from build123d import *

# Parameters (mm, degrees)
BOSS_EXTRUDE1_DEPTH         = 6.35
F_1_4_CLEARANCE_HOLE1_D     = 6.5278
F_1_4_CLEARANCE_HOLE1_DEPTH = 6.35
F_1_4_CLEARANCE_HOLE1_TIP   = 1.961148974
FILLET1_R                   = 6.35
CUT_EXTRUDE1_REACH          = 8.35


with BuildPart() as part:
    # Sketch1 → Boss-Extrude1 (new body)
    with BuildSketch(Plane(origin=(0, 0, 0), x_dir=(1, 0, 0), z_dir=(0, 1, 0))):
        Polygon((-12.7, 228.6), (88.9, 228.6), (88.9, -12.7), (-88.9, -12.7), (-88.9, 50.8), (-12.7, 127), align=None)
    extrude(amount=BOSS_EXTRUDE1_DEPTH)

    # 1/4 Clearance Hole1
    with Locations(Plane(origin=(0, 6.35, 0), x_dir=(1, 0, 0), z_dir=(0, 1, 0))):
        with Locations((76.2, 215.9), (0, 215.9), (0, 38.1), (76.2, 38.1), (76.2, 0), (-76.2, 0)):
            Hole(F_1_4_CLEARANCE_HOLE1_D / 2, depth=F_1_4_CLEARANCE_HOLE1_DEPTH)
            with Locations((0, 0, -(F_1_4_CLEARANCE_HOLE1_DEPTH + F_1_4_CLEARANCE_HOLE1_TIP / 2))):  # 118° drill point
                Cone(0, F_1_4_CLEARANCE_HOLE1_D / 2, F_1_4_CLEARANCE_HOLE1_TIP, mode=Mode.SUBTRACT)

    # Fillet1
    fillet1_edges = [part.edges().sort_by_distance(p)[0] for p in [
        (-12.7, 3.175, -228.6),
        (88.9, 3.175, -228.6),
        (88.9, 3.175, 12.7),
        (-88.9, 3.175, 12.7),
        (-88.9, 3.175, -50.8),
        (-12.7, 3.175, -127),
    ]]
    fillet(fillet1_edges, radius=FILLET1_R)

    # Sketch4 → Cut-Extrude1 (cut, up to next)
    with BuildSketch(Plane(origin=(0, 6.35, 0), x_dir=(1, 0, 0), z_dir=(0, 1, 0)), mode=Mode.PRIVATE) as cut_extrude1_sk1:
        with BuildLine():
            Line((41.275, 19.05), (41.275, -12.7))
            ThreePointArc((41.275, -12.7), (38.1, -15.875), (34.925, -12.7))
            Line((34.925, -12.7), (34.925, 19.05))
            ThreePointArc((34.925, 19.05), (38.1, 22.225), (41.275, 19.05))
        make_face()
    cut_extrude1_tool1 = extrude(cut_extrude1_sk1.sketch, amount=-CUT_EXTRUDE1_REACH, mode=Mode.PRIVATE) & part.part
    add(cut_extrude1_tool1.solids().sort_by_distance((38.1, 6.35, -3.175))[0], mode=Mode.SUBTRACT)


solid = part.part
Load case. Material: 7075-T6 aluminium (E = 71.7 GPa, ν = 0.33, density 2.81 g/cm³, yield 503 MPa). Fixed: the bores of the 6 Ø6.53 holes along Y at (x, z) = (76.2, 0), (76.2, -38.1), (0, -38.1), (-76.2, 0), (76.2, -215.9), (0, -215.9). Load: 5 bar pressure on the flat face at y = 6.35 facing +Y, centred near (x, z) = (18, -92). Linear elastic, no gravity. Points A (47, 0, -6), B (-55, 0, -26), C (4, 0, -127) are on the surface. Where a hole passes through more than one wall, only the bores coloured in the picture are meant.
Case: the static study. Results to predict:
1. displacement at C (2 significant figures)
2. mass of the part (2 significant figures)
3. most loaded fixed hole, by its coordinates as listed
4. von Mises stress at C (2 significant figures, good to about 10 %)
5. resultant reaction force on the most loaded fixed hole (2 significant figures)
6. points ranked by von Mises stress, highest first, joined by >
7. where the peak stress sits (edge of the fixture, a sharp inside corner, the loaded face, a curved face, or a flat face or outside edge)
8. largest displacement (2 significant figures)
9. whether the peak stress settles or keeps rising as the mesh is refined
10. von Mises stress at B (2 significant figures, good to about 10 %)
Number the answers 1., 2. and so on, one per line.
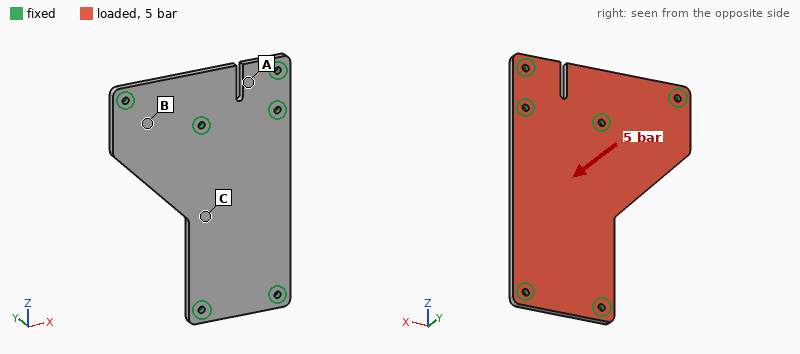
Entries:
1. 1.0 mm
2. 570 g
3. (0, -38.1)
4. 110 MPa
5. 5.9 kN
6. C > B > A
7. edge of the fixture
8. 1.1 mm
9. keeps rising
10. 63 MPa
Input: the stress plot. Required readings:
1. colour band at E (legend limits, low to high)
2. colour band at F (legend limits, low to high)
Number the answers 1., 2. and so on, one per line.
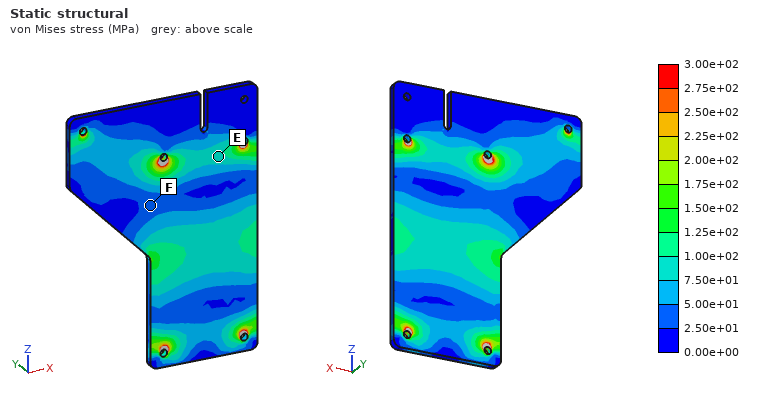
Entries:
1. 7.50e+01 to 1.00e+02 MPa
2. 2.50e+01 to 5.00e+01 MPa
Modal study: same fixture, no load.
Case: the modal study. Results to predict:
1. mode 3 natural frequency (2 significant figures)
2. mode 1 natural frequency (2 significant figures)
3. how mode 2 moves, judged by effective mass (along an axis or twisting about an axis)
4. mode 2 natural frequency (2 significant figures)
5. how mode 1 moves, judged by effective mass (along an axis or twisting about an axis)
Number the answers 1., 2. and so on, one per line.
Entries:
1. 2000 Hz
2. 950 Hz
3. twisting about Z
4. 1300 Hz
5. along Y
